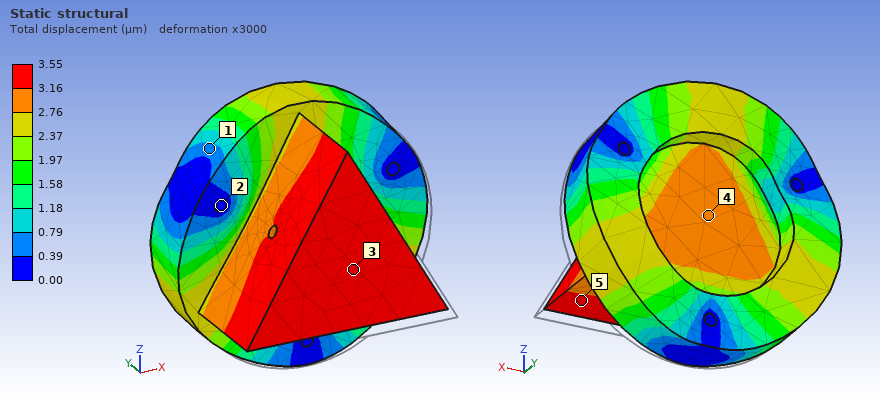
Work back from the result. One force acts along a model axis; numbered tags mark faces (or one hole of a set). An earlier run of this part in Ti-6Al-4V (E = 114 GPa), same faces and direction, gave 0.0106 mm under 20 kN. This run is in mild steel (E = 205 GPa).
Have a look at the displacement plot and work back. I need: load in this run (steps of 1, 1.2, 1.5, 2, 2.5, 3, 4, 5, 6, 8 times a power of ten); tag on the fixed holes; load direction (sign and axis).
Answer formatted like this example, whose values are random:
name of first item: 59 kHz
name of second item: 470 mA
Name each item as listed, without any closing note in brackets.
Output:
load in this run: 12 kN
tag on the fixed holes: 2
load direction: +Y
